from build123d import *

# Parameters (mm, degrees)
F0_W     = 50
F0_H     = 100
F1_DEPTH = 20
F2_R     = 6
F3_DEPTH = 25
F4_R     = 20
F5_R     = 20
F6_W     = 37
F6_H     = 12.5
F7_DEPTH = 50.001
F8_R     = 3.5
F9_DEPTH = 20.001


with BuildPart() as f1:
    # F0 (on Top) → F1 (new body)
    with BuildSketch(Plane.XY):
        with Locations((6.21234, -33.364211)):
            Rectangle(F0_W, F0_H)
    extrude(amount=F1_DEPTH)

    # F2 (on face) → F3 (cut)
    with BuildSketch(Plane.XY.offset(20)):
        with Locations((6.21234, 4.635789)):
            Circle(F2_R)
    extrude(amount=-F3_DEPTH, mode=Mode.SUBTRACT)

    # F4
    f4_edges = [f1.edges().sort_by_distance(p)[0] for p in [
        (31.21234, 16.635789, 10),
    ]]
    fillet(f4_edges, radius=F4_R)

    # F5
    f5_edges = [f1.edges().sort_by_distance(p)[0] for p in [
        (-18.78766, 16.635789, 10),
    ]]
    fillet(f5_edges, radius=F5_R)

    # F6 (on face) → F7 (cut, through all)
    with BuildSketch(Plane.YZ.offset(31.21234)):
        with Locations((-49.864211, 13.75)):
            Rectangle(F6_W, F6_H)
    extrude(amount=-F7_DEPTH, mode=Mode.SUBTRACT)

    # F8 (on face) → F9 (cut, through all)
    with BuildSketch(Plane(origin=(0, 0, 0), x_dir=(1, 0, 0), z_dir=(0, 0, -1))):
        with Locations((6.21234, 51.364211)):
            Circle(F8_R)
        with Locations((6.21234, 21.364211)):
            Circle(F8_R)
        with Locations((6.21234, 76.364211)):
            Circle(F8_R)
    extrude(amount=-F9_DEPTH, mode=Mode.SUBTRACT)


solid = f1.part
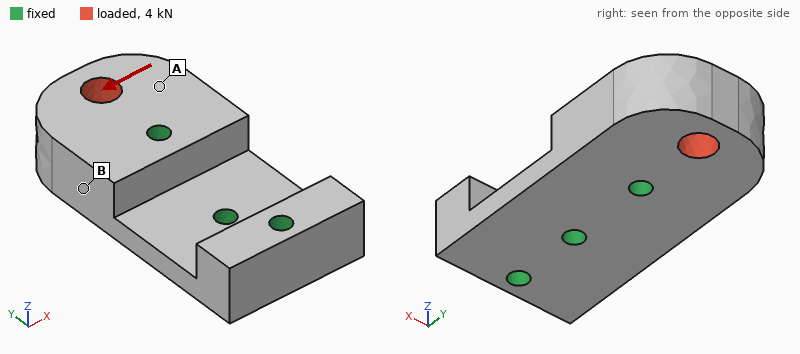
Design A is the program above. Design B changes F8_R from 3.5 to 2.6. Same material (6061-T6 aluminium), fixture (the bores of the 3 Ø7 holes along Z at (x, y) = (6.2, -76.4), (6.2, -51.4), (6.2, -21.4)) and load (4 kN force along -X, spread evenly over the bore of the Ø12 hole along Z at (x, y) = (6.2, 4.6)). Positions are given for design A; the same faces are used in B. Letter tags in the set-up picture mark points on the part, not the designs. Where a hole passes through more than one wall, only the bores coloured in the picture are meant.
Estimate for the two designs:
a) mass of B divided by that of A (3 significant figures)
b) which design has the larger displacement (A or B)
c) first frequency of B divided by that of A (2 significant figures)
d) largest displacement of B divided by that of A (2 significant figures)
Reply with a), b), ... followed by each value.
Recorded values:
a) 1.01
b) B
c) 0.92
d) 1.2
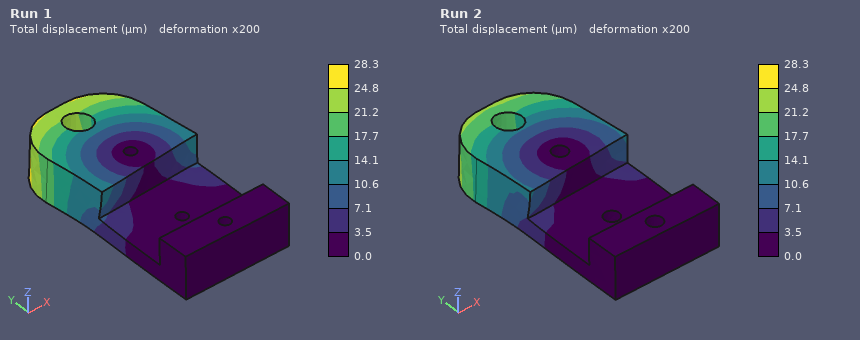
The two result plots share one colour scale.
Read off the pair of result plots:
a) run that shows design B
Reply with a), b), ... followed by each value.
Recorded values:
a) Run 1
